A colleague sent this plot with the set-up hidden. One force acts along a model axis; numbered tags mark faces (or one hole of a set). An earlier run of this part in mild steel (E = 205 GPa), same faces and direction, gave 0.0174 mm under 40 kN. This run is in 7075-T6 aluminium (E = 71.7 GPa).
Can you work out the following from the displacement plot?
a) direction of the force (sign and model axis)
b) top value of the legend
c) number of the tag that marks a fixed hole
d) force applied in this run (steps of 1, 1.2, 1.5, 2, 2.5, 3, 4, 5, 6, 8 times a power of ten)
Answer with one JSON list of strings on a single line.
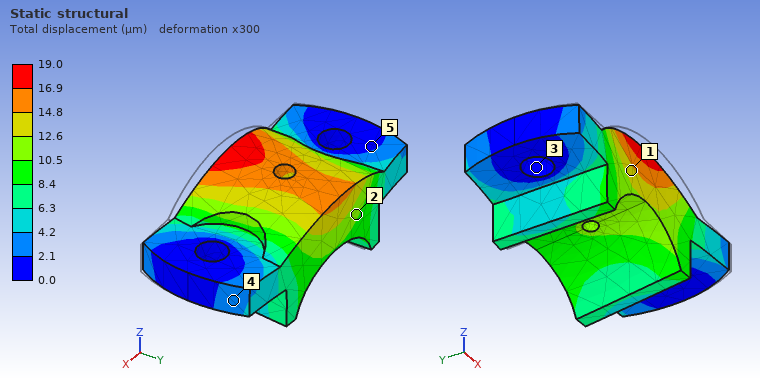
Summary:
["+Y", "19.0 µm", "3", "15 kN"]
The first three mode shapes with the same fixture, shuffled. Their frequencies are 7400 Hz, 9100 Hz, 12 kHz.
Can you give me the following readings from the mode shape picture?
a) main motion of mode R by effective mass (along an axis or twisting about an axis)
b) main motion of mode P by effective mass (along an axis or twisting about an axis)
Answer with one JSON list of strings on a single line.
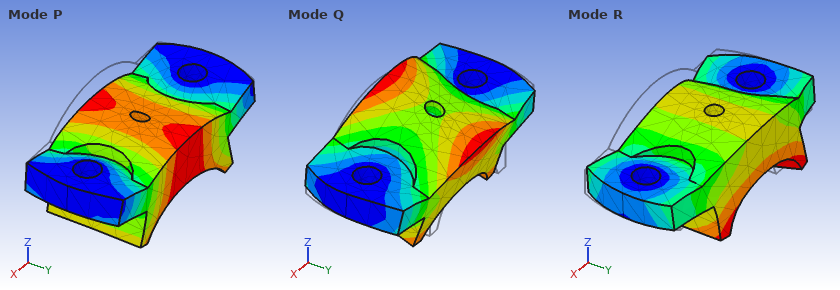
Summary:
["along Y", "along Z"]
